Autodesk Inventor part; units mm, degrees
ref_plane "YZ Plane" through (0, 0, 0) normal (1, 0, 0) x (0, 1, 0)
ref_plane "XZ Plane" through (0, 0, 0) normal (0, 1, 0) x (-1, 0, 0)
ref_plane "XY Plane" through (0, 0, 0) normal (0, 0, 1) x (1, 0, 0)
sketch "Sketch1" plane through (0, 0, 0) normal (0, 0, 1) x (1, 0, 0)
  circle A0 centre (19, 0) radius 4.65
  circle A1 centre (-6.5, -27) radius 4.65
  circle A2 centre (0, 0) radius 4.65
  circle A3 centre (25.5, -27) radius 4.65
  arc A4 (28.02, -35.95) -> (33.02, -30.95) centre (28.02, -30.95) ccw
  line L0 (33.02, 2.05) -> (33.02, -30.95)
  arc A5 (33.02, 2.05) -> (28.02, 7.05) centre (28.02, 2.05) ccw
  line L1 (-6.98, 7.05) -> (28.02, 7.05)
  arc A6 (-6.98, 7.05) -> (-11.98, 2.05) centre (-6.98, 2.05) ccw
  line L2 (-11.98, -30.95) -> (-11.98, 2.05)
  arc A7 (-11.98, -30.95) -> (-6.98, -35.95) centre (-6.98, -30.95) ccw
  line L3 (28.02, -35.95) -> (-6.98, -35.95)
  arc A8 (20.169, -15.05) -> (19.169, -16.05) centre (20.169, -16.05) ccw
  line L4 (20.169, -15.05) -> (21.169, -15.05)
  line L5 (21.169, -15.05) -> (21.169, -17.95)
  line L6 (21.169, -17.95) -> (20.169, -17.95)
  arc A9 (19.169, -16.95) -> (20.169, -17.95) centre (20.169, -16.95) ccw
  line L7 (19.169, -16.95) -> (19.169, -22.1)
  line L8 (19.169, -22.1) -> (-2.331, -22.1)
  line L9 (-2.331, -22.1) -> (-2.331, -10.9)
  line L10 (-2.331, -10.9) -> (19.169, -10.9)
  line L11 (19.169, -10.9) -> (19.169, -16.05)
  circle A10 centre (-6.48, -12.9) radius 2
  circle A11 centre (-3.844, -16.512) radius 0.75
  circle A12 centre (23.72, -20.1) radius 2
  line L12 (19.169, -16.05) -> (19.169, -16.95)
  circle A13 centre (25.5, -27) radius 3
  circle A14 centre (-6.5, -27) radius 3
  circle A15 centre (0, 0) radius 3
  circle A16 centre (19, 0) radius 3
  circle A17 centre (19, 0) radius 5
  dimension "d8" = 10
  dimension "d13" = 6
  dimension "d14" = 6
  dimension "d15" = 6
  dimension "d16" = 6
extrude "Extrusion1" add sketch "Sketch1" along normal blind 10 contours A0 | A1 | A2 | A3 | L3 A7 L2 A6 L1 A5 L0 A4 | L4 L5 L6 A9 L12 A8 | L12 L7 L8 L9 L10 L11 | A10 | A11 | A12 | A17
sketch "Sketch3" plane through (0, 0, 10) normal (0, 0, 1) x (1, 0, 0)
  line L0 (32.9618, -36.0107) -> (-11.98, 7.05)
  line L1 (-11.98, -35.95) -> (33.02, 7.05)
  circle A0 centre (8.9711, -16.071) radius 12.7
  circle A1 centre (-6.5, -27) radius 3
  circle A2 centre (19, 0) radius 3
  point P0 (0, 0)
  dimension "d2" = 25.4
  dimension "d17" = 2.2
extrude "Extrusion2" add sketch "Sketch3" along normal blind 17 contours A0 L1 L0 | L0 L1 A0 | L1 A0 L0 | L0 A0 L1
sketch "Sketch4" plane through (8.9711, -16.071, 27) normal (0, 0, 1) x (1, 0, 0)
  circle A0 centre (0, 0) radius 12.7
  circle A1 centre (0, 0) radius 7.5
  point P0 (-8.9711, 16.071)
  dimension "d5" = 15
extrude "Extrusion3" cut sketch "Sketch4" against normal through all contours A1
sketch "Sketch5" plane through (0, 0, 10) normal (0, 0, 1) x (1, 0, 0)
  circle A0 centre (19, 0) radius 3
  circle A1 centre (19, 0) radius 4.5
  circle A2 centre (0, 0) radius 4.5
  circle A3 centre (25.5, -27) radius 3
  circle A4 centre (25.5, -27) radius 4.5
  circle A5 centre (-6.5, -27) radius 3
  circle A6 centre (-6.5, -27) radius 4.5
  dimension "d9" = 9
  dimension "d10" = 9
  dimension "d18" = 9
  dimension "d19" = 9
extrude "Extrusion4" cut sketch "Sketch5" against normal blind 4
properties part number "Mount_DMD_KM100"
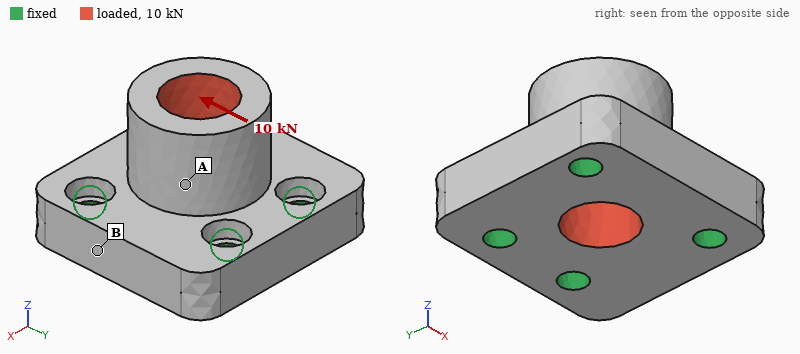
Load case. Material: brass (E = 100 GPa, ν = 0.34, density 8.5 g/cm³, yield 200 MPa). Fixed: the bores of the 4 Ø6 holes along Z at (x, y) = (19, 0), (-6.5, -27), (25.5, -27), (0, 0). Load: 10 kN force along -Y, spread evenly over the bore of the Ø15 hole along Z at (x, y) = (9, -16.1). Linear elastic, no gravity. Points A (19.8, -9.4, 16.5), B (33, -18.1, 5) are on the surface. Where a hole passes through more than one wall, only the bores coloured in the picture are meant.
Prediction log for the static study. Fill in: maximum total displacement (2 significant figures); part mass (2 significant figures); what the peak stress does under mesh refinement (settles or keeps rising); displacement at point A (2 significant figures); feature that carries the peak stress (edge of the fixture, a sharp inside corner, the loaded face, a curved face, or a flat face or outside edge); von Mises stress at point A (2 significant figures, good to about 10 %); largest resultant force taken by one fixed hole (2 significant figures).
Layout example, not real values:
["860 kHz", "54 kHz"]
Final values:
["24 µm", "180 g", "keeps rising", "12 µm", "edge of the fixture", "25 MPa", "3.4 kN"]
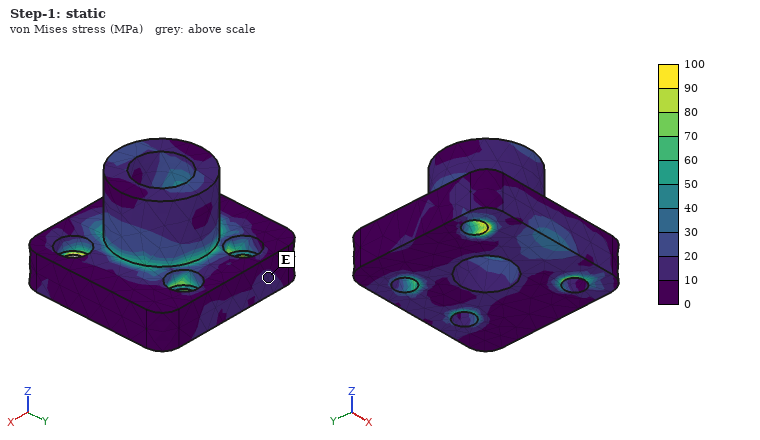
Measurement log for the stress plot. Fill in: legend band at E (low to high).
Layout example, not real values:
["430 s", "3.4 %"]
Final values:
["10 to 20 MPa"]
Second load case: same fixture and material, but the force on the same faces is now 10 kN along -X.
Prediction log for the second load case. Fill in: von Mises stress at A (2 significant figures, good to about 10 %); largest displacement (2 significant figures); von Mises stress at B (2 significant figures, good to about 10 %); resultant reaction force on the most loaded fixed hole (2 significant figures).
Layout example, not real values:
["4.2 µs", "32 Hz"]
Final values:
["18 MPa", "22 µm", "16 MPa", "3.8 kN"]
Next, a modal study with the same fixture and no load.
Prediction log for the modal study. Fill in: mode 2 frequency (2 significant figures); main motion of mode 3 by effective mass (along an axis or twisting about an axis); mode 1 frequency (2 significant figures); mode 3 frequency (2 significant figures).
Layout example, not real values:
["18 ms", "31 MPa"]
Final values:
["14 kHz", "along Z", "13 kHz", "19 kHz"]
